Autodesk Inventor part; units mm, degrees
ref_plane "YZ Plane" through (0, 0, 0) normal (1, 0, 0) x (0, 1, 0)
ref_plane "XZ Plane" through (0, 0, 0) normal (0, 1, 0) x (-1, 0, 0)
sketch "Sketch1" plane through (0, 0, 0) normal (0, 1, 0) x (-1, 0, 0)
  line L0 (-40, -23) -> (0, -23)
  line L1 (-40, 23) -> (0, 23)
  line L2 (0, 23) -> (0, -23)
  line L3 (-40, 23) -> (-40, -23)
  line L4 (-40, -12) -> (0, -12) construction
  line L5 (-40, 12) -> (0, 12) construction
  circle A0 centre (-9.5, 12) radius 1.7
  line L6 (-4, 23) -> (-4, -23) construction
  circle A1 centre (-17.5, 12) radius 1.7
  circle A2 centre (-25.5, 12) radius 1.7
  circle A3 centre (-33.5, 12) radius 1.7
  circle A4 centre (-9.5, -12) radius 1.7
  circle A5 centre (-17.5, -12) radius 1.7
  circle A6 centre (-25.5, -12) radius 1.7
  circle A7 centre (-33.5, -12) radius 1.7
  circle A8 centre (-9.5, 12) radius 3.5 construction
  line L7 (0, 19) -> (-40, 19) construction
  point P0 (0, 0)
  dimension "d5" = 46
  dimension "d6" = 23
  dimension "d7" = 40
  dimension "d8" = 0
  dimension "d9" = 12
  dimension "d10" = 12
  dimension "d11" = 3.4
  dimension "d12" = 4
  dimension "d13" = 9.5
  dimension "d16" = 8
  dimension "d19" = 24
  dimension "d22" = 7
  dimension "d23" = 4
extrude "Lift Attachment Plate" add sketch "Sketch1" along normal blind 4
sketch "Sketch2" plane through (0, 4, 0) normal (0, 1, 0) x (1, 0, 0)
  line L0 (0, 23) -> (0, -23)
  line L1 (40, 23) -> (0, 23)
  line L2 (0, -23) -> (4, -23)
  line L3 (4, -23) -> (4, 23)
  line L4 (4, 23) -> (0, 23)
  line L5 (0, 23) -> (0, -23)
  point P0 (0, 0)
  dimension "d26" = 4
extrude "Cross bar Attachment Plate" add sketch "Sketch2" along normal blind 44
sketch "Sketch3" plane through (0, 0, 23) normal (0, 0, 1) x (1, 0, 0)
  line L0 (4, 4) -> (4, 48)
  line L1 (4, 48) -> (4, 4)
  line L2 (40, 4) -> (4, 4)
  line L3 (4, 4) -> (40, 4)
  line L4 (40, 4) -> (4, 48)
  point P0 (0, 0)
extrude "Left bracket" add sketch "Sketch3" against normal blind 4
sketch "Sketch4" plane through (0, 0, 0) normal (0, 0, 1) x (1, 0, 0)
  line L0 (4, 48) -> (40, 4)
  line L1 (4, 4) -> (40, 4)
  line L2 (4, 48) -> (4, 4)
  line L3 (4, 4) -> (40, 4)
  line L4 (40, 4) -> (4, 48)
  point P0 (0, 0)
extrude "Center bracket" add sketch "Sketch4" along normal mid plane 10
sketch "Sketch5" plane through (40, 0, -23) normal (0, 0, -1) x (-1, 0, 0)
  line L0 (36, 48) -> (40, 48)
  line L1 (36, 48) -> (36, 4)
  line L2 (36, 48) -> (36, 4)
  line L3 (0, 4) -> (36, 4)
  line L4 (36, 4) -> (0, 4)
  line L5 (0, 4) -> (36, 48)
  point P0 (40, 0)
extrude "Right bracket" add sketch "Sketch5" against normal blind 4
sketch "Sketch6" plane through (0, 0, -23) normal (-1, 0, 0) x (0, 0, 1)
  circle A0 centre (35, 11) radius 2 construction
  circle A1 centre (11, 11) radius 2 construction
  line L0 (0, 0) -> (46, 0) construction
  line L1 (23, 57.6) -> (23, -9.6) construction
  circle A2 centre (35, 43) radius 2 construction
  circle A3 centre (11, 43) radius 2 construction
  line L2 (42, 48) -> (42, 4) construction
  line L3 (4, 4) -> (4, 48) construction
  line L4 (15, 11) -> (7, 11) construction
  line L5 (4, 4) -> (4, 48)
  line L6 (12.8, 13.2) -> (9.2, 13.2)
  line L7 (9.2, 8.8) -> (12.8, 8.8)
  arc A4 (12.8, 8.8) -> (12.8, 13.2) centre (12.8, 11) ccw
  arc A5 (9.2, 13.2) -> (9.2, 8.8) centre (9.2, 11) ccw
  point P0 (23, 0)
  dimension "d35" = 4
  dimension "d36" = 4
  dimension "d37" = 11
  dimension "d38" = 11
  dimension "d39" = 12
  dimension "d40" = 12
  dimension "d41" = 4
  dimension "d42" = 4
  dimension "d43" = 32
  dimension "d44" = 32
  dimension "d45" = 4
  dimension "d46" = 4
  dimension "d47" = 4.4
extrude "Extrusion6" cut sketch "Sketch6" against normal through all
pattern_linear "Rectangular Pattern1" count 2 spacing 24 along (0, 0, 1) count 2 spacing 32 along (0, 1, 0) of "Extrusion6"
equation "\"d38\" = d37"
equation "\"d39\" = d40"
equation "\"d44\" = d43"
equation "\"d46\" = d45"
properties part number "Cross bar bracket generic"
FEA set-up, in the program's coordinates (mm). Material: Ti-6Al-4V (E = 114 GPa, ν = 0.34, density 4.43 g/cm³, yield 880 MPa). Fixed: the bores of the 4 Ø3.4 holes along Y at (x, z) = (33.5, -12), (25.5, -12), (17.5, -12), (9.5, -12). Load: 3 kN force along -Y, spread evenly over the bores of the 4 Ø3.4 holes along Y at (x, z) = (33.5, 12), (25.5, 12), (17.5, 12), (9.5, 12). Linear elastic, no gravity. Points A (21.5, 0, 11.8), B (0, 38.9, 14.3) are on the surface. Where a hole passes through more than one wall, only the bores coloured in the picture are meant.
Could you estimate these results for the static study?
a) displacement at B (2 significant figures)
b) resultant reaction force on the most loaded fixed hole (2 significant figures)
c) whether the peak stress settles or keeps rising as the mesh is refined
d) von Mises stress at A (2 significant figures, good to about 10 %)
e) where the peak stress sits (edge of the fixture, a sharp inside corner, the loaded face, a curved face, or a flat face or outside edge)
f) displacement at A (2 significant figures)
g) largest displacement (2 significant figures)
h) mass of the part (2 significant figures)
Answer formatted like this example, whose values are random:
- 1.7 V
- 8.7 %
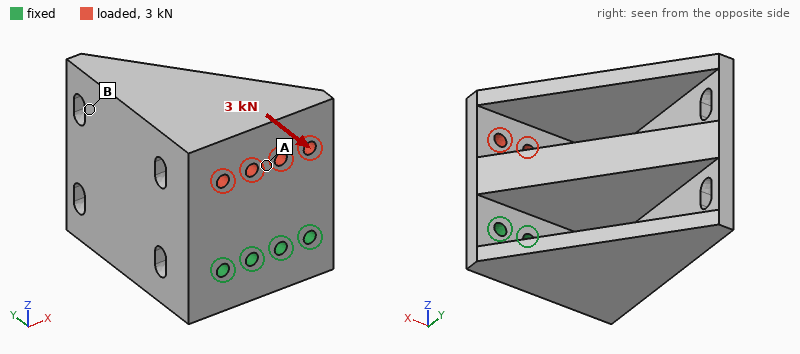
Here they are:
- 0.33 mm
- 840 N
- keeps rising
- 100 MPa
- edge of the fixture
- 0.19 mm
- 0.42 mm
- 130 g
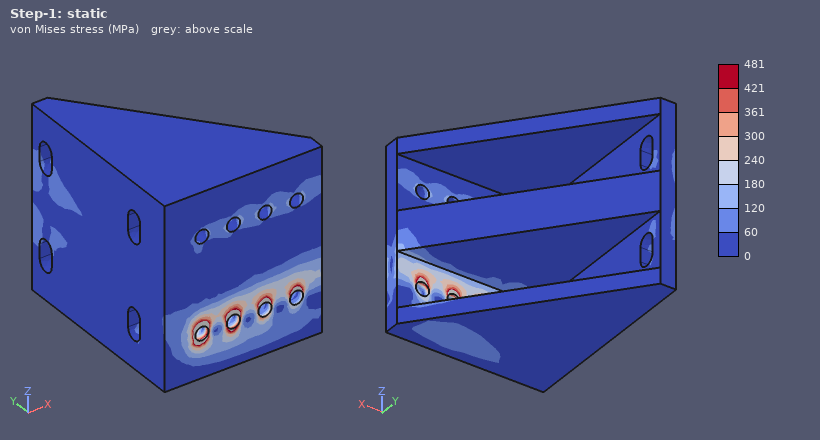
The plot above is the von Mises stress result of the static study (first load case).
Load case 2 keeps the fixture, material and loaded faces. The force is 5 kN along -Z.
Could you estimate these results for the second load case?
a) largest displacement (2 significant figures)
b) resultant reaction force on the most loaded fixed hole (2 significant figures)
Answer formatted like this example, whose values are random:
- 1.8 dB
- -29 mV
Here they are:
- 8.5 µm
- 1.5 kN
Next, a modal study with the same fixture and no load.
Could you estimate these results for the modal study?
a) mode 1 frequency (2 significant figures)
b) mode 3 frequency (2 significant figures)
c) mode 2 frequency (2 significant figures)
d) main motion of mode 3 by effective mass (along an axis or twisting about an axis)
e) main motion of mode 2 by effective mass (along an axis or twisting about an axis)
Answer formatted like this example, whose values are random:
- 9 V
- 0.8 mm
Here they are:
- 1600 Hz
- 6800 Hz
- 3900 Hz
- along Y
- along X
